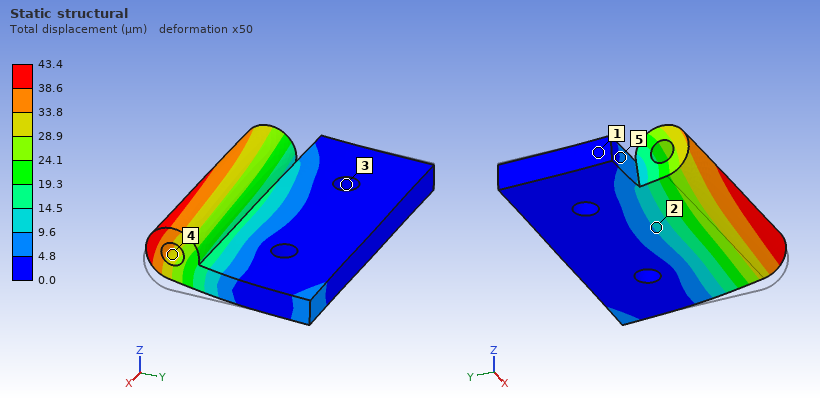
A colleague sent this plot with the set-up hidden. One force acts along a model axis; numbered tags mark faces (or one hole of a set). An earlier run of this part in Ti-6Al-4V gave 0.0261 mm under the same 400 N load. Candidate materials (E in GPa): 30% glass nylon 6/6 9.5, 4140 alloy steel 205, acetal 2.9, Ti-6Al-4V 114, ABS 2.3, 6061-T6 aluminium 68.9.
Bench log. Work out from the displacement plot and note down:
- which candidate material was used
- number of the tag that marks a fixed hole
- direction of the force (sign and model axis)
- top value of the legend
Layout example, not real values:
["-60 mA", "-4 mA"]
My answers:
["6061-T6 aluminium", "3", "+Z", "43.4 µm"]
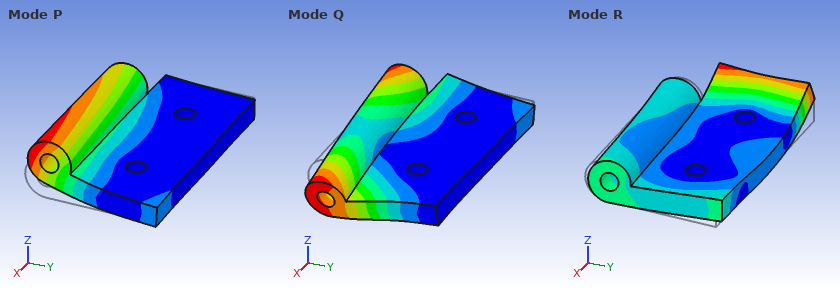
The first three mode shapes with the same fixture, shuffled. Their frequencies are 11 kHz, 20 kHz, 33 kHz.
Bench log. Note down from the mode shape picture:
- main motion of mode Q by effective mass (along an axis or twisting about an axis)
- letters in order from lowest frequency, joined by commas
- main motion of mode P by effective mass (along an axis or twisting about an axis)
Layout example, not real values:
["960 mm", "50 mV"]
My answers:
["twisting about Y", "P, Q, R", "along Z"]
